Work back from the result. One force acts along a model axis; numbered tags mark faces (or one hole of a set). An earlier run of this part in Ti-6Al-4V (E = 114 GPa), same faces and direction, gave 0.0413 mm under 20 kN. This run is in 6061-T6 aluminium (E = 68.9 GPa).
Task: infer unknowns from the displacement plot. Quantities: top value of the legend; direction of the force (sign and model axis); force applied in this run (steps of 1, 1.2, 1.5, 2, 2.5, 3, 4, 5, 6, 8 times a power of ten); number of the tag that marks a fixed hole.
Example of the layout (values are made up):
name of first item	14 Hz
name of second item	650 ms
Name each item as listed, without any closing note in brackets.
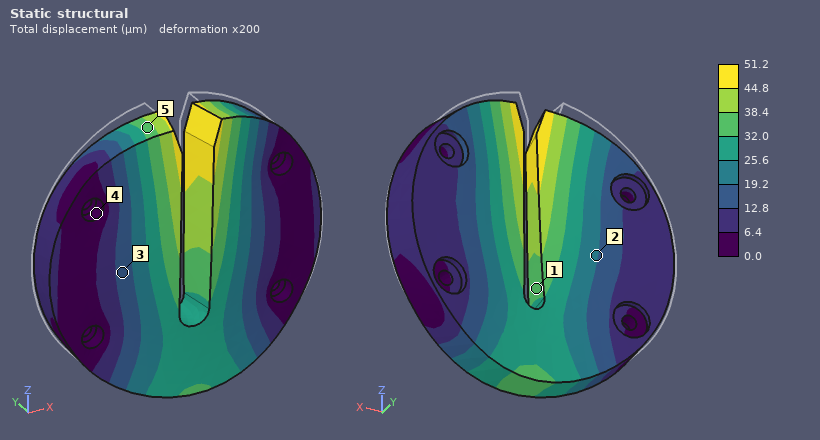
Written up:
top value of the legend	51.2 µm
direction of the force	-Y
force applied in this run	15 kN
number of the tag that marks a fixed hole	4
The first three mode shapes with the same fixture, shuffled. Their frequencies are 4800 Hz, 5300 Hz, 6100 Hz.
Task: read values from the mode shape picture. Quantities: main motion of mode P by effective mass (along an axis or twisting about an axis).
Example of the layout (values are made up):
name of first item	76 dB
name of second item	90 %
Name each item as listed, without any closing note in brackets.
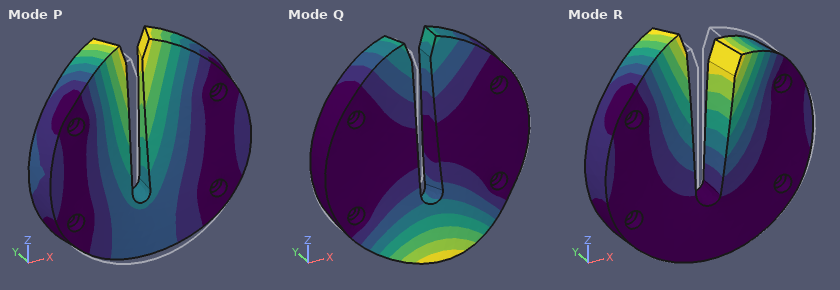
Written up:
main motion of mode P by effective mass	along Y
